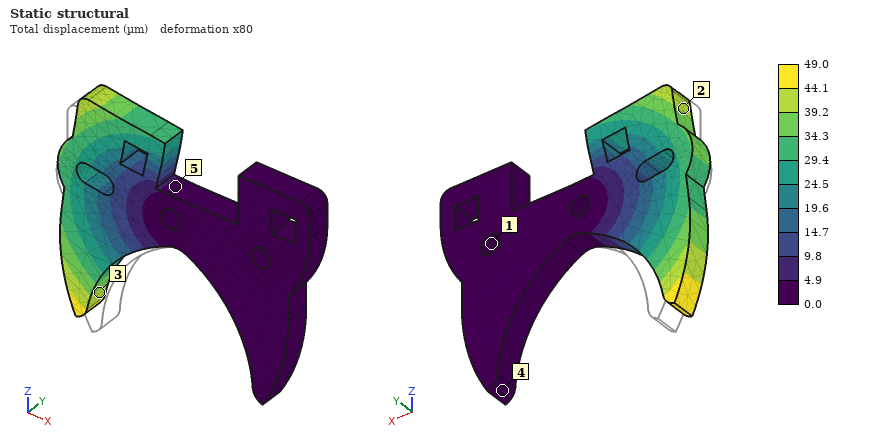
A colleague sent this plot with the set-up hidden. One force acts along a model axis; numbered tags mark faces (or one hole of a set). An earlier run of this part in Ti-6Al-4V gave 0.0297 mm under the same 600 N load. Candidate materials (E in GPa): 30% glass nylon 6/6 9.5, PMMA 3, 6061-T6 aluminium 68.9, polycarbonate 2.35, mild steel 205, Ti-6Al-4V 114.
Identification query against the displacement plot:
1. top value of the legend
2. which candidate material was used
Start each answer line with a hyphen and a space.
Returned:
- 49.0 µm
- 6061-T6 aluminium
